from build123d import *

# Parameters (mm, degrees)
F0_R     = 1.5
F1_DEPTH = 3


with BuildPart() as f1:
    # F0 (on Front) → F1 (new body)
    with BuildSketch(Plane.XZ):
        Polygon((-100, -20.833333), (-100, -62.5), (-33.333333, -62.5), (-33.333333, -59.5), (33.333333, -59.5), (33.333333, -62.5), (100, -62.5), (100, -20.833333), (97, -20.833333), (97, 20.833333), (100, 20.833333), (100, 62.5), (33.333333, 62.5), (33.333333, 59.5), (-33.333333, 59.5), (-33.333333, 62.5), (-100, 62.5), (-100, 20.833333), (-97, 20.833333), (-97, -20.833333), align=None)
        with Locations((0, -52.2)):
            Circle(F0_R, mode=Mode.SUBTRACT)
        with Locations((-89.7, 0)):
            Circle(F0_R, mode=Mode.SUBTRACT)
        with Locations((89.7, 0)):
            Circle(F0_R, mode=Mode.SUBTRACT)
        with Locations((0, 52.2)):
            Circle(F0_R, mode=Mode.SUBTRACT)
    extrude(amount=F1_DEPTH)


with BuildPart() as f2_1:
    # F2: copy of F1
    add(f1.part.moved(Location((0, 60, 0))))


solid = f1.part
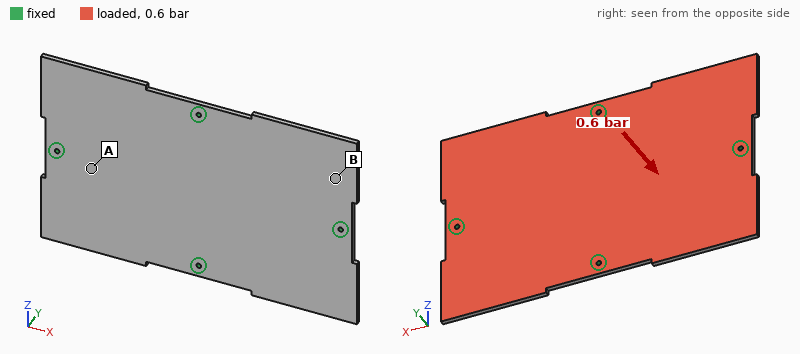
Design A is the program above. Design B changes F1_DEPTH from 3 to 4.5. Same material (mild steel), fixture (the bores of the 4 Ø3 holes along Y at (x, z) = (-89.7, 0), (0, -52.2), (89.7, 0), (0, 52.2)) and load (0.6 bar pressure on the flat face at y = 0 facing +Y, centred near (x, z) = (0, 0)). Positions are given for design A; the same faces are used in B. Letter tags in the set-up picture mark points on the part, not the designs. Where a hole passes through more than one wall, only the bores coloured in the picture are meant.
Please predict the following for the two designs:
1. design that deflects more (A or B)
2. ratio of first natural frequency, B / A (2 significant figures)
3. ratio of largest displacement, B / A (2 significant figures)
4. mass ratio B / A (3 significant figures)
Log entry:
A
1.4
0.30
1.50
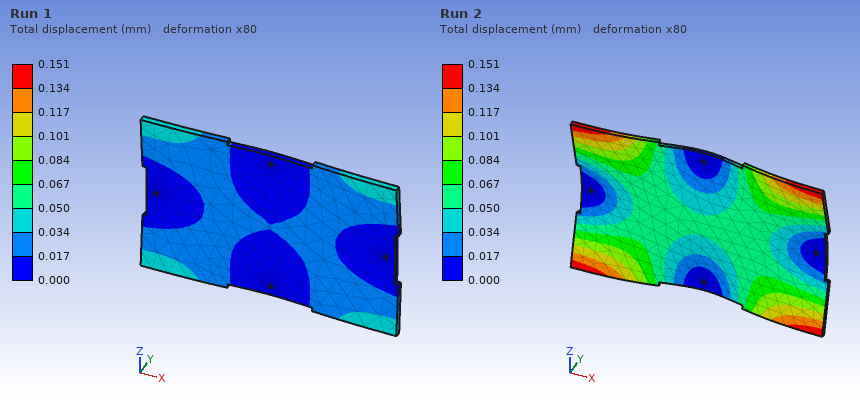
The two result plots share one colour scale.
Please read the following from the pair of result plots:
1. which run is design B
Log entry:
Run 1
